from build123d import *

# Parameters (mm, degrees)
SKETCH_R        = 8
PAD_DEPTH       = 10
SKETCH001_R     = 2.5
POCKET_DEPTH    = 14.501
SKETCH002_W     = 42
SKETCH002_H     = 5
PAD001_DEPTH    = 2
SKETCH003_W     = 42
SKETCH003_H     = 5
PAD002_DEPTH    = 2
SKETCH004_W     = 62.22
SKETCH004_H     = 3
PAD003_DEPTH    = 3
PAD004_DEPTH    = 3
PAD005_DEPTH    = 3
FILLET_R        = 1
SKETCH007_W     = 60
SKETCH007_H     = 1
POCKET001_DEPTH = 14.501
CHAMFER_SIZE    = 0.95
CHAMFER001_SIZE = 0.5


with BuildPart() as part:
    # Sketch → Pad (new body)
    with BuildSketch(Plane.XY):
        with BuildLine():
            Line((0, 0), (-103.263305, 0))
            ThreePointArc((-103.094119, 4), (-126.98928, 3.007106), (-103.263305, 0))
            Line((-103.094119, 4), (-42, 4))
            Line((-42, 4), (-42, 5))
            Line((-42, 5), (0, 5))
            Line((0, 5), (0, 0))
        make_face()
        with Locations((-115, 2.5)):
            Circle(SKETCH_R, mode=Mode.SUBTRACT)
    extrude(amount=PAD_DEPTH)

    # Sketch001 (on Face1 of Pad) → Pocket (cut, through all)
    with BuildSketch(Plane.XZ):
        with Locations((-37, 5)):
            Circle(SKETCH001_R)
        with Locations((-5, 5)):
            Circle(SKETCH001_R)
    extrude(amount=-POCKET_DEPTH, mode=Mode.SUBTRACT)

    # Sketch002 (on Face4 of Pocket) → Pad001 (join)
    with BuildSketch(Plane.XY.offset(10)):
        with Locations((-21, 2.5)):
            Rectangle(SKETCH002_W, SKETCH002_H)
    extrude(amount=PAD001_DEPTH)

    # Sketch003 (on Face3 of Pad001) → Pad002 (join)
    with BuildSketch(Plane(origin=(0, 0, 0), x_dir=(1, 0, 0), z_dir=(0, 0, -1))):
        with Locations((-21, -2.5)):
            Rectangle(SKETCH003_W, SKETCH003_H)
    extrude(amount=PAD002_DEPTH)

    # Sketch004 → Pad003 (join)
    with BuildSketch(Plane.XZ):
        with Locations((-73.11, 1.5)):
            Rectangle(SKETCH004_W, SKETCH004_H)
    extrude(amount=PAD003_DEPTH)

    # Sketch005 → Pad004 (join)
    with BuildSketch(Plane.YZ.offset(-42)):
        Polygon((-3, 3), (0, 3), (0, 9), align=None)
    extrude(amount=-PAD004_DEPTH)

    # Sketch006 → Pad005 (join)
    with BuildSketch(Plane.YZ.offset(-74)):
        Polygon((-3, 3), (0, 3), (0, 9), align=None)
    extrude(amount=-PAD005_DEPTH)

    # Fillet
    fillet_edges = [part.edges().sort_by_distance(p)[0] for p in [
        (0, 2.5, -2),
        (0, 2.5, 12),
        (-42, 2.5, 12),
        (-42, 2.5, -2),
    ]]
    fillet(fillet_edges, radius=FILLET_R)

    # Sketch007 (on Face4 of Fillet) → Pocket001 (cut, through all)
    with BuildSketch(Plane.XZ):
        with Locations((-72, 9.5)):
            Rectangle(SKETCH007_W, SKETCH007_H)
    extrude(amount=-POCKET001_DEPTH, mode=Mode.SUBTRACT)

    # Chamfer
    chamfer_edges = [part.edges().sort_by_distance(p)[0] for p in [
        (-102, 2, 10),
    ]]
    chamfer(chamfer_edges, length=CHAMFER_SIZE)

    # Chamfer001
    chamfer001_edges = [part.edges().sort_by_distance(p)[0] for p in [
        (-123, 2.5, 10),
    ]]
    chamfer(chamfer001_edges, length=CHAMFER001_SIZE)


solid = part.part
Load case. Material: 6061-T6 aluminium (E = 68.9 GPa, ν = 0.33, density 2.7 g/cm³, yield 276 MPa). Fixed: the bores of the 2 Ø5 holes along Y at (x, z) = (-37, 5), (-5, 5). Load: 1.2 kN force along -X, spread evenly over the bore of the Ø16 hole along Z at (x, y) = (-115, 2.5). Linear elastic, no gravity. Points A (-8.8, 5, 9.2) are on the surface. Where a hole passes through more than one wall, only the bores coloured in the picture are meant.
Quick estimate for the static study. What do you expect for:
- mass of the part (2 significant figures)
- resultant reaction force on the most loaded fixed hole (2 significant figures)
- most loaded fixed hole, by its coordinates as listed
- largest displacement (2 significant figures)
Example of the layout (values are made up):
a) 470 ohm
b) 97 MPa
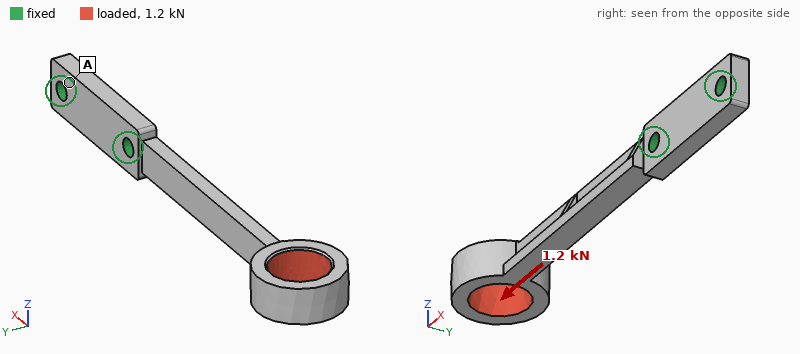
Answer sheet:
a) 22 g
b) 1.2 kN
c) (-37, 5)
d) 0.51 mm
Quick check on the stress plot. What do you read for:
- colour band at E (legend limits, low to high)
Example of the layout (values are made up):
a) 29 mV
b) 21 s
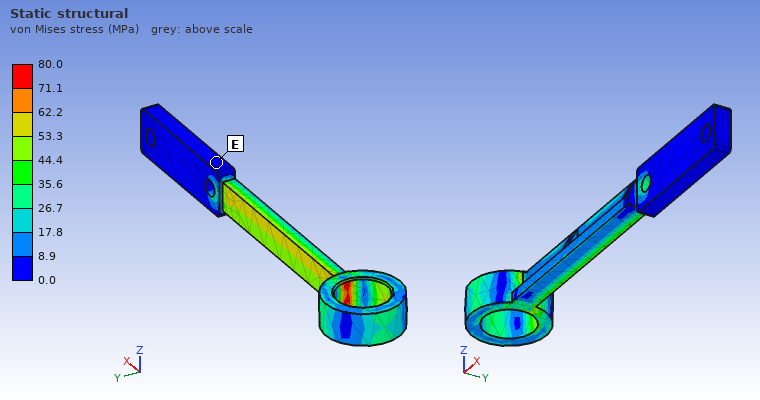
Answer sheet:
a) 0.0 to 8.9 MPa
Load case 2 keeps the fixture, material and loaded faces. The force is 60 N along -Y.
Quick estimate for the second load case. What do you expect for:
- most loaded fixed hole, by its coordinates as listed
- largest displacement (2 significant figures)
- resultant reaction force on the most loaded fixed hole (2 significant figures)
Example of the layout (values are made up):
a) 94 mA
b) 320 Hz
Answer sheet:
a) (-37, 5)
b) 1.5 mm
c) 64 N
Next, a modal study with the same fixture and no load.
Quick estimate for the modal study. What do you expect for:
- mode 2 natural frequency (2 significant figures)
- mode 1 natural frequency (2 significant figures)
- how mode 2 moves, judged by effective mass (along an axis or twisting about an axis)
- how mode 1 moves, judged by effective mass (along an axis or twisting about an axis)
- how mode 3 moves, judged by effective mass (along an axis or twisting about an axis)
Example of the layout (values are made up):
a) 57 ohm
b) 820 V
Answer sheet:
a) 660 Hz
b) 390 Hz
c) along Z
d) along Y
e) twisting about X
